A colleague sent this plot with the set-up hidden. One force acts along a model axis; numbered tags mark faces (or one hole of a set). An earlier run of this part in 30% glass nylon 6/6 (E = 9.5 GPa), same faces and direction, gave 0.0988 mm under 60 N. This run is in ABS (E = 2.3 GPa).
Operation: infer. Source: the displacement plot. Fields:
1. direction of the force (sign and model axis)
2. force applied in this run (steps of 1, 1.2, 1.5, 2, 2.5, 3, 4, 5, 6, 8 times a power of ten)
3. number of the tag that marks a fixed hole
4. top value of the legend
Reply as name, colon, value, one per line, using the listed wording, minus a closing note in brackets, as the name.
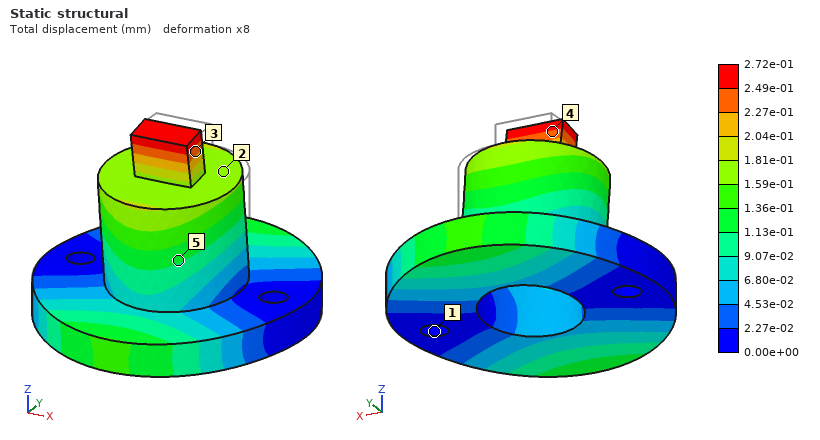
direction of the force: -Y
force applied in this run: 40 N
number of the tag that marks a fixed hole: 1
top value of the legend: 2.72e-01 mm
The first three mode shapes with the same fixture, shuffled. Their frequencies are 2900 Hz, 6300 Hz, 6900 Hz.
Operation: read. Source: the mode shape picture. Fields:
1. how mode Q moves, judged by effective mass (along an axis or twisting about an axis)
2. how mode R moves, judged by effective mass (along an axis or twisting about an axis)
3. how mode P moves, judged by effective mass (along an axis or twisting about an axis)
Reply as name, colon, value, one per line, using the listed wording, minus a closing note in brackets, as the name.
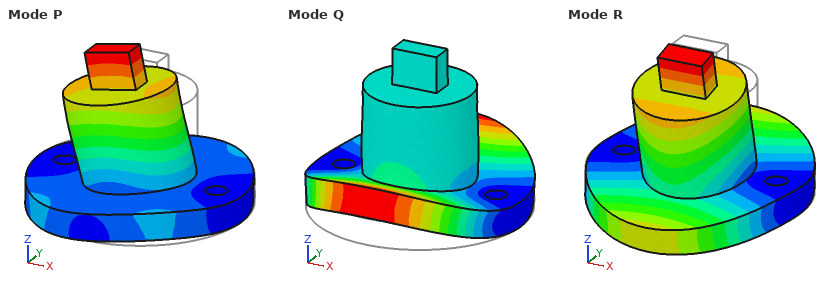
how mode Q moves, judged by effective mass: along Z
how mode R moves, judged by effective mass: along Y
how mode P moves, judged by effective mass: along X
